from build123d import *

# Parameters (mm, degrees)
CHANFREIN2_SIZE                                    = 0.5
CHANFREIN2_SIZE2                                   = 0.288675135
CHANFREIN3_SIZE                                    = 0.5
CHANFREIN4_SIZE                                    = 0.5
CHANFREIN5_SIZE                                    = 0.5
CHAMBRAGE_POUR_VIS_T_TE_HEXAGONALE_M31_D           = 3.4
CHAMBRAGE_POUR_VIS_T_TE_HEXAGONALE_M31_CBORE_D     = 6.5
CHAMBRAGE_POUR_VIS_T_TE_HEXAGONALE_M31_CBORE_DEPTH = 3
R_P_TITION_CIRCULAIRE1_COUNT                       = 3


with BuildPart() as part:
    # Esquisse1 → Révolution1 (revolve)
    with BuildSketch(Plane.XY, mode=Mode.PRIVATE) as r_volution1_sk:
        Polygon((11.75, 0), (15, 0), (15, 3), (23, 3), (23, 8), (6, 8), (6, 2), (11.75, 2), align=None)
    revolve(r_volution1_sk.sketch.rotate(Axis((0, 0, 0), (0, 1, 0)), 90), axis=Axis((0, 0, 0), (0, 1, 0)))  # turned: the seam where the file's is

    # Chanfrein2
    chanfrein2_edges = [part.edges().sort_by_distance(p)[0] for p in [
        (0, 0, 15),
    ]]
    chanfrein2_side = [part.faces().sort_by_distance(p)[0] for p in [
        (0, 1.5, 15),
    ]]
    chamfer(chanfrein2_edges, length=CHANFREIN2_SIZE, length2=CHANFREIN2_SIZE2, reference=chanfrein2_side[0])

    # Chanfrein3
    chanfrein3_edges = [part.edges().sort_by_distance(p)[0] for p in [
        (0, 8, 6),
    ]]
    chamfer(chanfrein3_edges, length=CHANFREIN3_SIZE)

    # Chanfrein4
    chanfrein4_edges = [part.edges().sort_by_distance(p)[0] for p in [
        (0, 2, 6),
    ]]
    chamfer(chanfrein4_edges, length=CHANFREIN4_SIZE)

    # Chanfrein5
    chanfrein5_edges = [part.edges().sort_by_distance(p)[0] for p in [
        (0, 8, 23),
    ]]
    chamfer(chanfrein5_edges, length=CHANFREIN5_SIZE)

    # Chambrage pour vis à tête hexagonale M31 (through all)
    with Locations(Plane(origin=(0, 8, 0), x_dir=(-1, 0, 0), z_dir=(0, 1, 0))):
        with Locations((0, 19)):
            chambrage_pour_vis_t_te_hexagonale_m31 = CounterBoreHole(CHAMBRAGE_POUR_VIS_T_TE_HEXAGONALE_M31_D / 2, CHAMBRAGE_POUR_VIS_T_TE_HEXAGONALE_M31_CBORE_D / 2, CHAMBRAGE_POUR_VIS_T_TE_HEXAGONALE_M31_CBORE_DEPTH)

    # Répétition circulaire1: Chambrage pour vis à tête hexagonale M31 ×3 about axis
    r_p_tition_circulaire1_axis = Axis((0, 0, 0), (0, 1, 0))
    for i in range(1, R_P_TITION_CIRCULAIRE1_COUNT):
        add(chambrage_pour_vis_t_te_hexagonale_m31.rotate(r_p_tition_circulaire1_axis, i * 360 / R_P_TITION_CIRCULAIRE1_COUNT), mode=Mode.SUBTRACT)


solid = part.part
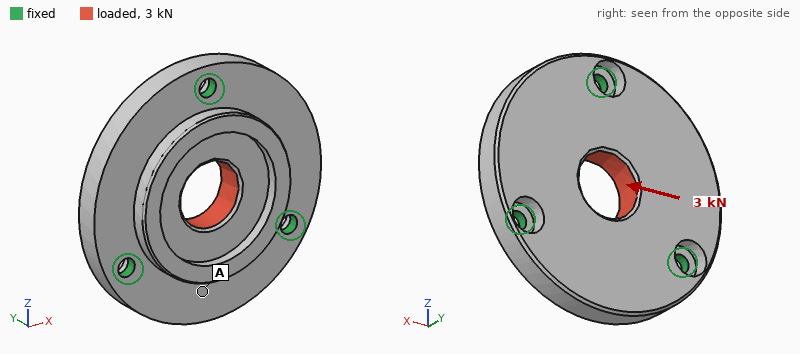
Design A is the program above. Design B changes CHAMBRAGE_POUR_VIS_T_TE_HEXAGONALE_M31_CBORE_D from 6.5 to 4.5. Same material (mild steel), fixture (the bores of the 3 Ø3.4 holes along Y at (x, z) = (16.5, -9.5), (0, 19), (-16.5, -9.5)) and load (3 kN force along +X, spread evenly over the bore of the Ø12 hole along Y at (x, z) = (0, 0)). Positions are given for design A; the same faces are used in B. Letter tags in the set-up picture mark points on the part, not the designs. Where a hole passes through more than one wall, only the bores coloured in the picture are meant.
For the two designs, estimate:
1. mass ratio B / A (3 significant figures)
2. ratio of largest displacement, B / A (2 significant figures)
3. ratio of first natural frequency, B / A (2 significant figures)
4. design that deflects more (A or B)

1.02
0.89
1.0
A
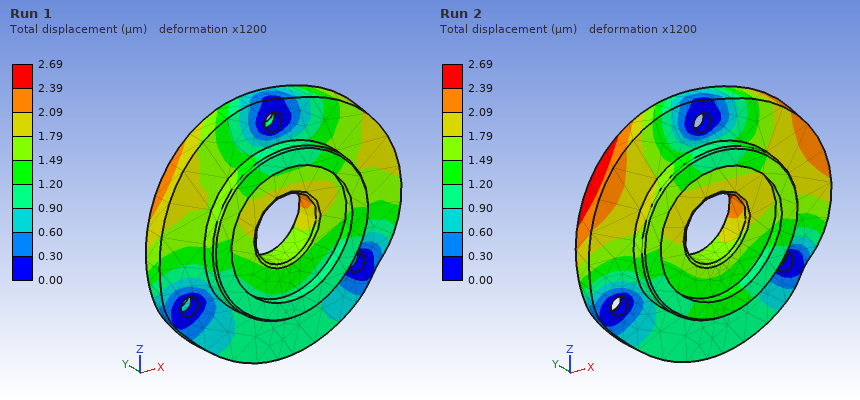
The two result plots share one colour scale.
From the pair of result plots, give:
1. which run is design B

Run 1
